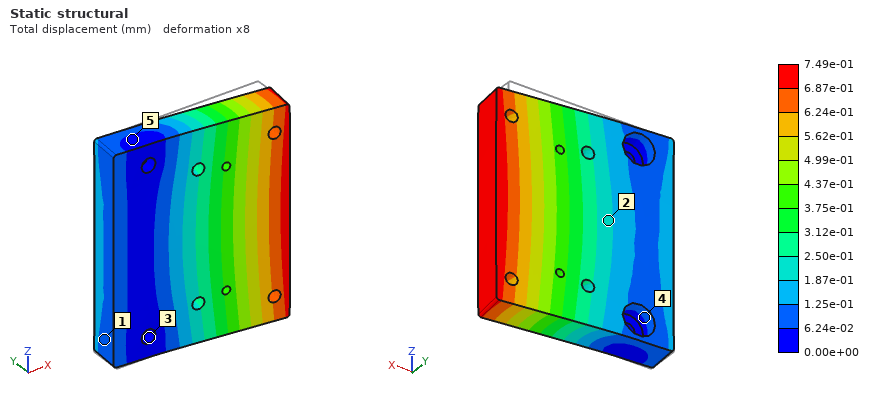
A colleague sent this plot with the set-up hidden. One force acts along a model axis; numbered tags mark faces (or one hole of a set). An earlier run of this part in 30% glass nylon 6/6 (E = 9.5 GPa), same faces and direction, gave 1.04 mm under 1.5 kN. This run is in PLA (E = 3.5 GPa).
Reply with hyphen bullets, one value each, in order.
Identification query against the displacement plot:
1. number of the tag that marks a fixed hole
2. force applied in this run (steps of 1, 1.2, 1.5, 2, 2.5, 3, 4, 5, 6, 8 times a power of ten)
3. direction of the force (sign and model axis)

- 3
- 400 N
- -Y
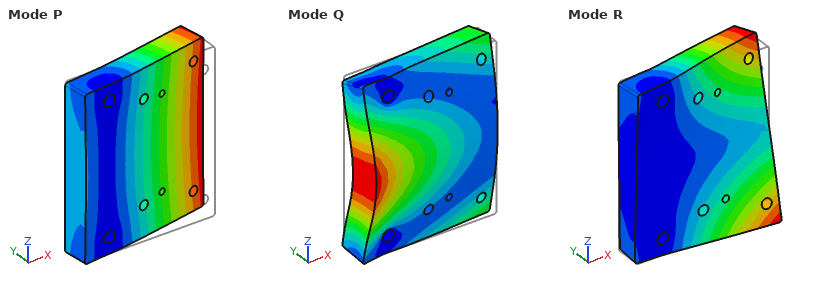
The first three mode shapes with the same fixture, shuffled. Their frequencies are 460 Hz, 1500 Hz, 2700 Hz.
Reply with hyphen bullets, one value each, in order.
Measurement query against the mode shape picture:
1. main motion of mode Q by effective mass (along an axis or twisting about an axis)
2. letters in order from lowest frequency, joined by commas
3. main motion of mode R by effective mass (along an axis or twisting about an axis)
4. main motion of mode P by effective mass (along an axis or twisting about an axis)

- along Y
- P, R, Q
- twisting about X
- along Y
